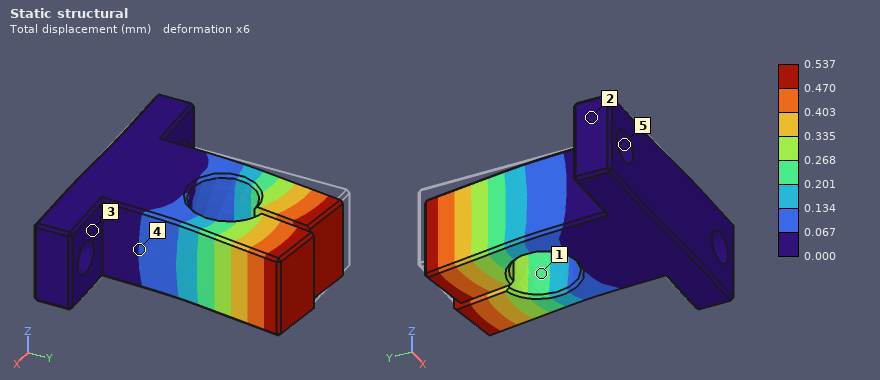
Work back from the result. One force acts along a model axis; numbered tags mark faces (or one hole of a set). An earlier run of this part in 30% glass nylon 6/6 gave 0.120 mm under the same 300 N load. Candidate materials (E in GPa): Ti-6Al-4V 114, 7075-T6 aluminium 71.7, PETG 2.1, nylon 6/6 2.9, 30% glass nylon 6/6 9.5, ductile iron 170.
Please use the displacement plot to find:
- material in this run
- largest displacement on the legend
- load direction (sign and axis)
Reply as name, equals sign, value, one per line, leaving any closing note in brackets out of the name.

material in this run = PETG
largest displacement on the legend = 0.537 mm
load direction = +X
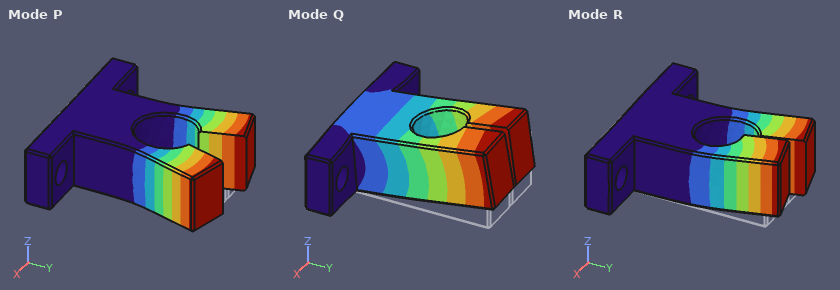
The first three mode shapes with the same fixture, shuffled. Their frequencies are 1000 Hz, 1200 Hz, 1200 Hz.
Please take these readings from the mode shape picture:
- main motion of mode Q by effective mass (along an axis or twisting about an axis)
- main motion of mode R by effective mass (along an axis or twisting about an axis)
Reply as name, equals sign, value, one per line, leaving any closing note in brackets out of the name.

main motion of mode Q by effective mass = along Z
main motion of mode R by effective mass = along X
